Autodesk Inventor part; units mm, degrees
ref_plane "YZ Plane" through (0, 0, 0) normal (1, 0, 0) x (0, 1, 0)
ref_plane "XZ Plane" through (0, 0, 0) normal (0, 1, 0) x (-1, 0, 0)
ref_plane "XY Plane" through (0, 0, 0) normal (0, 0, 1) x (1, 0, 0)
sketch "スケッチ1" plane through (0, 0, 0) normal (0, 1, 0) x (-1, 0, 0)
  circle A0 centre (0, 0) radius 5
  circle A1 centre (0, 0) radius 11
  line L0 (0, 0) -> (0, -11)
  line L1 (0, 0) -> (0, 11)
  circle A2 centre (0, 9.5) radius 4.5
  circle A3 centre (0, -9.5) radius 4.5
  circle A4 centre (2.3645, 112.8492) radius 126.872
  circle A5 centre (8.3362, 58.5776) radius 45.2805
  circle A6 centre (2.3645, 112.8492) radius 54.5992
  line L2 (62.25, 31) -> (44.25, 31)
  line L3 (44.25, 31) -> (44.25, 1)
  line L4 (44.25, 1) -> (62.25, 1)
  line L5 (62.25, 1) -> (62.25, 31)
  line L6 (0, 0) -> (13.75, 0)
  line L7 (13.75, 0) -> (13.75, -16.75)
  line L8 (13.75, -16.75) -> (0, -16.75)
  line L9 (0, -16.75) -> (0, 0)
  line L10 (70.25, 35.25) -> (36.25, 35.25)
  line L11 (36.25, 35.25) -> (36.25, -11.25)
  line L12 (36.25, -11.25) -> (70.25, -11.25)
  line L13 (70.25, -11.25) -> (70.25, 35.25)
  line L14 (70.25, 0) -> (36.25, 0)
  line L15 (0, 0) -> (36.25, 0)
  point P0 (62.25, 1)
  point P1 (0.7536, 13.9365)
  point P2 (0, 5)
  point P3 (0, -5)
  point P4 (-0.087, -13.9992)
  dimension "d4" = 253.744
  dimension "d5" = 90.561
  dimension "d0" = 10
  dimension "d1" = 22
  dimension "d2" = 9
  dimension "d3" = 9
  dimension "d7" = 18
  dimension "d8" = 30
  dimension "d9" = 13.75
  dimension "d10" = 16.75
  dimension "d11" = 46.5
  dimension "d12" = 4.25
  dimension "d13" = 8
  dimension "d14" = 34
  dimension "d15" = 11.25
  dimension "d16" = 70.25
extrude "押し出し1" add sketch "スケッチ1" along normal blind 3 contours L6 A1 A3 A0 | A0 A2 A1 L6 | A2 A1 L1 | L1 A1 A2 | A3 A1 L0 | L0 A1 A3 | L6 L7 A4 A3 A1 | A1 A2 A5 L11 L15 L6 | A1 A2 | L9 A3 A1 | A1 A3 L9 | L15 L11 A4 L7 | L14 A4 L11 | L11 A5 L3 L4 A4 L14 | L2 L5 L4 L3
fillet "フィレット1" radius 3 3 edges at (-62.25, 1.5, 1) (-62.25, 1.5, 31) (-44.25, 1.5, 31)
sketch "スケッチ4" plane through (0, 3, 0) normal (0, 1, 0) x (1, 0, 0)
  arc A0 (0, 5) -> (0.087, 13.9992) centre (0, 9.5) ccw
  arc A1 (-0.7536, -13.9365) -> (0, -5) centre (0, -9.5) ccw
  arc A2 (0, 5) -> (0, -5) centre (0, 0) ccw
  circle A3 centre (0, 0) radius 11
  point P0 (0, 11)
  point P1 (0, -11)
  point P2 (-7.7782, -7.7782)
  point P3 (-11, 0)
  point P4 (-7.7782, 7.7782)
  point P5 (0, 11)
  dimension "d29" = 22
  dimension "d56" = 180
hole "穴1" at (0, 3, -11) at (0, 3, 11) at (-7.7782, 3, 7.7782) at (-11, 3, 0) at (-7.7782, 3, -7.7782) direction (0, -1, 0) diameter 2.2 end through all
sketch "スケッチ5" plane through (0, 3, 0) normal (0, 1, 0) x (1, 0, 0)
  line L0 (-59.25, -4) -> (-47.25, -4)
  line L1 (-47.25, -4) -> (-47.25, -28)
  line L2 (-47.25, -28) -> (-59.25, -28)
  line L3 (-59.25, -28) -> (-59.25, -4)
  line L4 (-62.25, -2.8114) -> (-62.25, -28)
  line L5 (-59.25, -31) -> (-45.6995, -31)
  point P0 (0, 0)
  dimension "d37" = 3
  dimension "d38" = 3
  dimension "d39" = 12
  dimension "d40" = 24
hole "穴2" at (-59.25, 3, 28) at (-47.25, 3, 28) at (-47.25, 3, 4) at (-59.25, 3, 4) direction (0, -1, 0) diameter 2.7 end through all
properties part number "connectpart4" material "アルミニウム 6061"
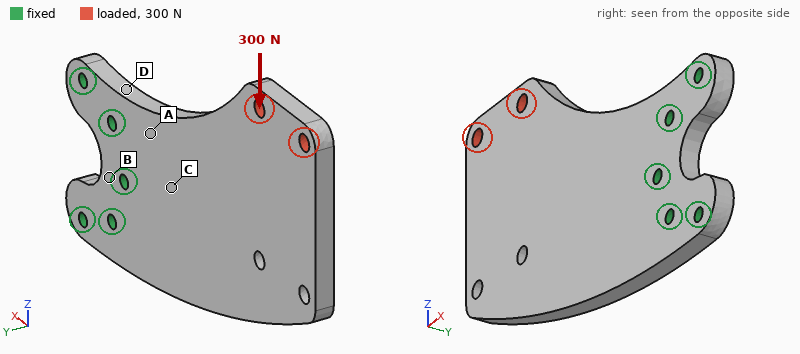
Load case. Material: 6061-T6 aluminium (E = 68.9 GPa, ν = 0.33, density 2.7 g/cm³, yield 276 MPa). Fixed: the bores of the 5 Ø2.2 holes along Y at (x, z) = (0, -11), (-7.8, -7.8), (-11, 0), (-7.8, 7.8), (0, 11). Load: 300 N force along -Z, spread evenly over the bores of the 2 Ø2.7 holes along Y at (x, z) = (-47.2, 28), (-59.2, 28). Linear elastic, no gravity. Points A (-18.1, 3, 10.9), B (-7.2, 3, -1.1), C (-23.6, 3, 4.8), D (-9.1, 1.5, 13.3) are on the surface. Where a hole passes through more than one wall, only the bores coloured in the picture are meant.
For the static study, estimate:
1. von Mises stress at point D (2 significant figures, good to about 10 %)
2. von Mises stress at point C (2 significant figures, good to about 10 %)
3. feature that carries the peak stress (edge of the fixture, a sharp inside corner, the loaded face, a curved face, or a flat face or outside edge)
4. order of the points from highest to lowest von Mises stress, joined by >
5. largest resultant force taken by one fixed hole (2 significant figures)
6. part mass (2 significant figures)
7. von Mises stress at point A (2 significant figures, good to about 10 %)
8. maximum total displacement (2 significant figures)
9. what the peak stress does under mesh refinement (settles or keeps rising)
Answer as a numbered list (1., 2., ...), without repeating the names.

1. 30 MPa
2. 10 MPa
3. edge of the fixture
4. D > A > C > B
5. 530 N
6. 15 g
7. 21 MPa
8. 56 µm
9. keeps rising
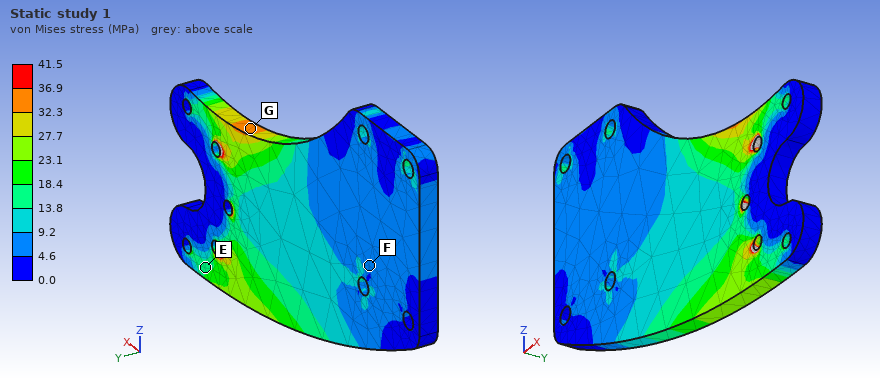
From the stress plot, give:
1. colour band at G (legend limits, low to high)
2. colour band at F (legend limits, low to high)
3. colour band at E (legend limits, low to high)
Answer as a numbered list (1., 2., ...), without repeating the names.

1. 32.3 to 36.9 MPa
2. 4.6 to 9.2 MPa
3. 13.8 to 18.4 MPa
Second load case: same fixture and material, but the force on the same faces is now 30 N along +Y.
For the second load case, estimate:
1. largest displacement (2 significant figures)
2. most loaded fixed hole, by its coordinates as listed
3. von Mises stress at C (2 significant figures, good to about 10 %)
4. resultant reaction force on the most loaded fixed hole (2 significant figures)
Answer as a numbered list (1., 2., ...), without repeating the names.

1. 0.38 mm
2. (-11, 0)
3. 25 MPa
4. 86 N
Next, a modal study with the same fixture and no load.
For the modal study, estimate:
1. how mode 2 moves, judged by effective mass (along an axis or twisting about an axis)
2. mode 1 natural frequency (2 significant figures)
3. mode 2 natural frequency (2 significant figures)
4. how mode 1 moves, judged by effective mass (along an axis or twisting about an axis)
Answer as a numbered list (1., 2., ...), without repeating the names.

1. twisting about X
2. 780 Hz
3. 2600 Hz
4. along Y
